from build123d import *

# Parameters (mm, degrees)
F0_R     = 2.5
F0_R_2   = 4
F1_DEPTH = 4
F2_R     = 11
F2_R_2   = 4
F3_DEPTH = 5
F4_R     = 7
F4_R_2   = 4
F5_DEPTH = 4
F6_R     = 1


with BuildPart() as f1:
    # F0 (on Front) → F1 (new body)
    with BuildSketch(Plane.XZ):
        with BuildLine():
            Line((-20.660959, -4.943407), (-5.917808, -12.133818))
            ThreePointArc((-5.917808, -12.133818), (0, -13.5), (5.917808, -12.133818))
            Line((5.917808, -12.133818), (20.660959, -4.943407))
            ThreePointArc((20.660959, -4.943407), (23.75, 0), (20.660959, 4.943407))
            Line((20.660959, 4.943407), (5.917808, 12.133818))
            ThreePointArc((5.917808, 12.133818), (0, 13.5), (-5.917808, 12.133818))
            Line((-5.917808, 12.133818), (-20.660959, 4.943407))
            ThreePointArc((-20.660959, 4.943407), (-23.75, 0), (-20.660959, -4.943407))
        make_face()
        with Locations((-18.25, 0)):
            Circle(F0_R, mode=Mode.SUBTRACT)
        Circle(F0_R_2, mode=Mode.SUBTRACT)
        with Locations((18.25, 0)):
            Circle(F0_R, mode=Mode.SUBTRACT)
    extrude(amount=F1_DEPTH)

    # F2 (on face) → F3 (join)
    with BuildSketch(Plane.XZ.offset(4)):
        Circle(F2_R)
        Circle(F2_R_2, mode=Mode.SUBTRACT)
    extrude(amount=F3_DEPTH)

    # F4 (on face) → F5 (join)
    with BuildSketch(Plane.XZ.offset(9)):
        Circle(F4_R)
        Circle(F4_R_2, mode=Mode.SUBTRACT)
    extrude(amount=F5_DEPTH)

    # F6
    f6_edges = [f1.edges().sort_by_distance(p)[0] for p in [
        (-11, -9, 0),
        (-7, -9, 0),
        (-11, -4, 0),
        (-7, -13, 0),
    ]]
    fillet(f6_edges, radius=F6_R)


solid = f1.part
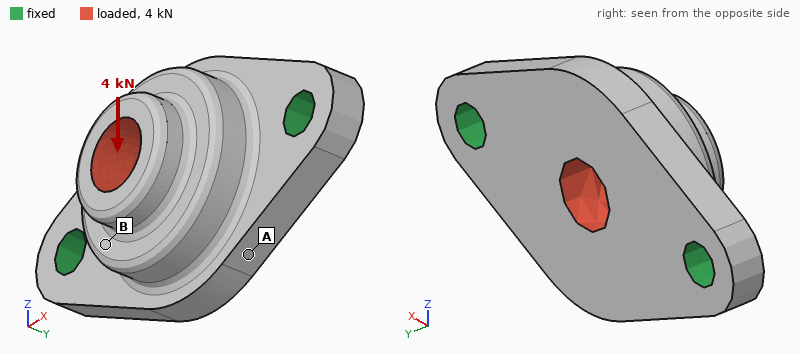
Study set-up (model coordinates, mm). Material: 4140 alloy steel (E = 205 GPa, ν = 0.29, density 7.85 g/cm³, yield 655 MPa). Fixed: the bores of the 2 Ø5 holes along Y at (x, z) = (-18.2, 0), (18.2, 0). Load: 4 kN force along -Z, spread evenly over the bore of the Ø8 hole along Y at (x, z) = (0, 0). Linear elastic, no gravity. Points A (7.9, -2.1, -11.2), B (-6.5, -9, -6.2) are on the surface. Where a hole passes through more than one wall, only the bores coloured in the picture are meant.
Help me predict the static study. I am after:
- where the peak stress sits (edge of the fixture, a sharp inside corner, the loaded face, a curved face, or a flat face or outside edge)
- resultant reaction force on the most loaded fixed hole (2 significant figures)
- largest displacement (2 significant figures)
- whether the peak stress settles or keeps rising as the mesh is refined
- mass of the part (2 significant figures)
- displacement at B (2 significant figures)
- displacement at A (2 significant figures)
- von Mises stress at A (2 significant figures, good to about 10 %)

edge of the fixture
2.0 kN
35 µm
keeps rising
40 g
26 µm
25 µm
57 MPa
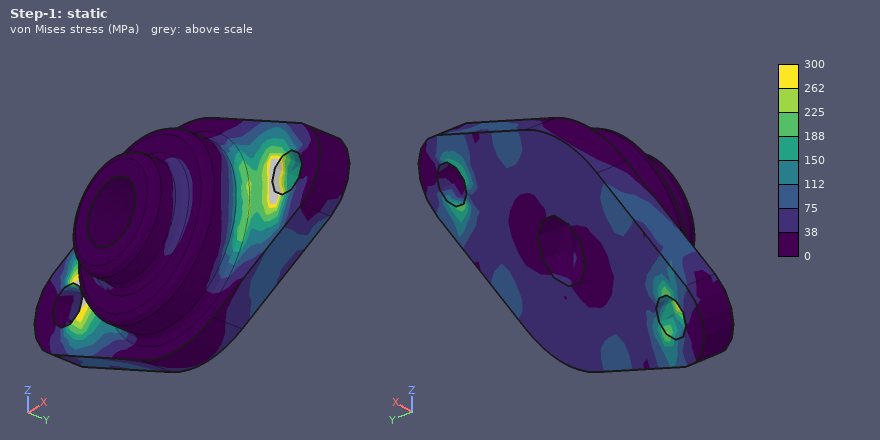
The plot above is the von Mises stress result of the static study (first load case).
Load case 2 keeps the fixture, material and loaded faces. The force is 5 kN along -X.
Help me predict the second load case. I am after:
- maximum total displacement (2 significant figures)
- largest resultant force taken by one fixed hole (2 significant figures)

6.7 µm
2.6 kN
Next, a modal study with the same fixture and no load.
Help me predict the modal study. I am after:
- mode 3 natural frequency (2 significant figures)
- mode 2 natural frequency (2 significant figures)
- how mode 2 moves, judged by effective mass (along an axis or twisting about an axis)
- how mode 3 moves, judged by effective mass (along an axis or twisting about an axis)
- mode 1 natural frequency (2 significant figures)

27 kHz
15 kHz
along Y
along Z
9900 Hz
